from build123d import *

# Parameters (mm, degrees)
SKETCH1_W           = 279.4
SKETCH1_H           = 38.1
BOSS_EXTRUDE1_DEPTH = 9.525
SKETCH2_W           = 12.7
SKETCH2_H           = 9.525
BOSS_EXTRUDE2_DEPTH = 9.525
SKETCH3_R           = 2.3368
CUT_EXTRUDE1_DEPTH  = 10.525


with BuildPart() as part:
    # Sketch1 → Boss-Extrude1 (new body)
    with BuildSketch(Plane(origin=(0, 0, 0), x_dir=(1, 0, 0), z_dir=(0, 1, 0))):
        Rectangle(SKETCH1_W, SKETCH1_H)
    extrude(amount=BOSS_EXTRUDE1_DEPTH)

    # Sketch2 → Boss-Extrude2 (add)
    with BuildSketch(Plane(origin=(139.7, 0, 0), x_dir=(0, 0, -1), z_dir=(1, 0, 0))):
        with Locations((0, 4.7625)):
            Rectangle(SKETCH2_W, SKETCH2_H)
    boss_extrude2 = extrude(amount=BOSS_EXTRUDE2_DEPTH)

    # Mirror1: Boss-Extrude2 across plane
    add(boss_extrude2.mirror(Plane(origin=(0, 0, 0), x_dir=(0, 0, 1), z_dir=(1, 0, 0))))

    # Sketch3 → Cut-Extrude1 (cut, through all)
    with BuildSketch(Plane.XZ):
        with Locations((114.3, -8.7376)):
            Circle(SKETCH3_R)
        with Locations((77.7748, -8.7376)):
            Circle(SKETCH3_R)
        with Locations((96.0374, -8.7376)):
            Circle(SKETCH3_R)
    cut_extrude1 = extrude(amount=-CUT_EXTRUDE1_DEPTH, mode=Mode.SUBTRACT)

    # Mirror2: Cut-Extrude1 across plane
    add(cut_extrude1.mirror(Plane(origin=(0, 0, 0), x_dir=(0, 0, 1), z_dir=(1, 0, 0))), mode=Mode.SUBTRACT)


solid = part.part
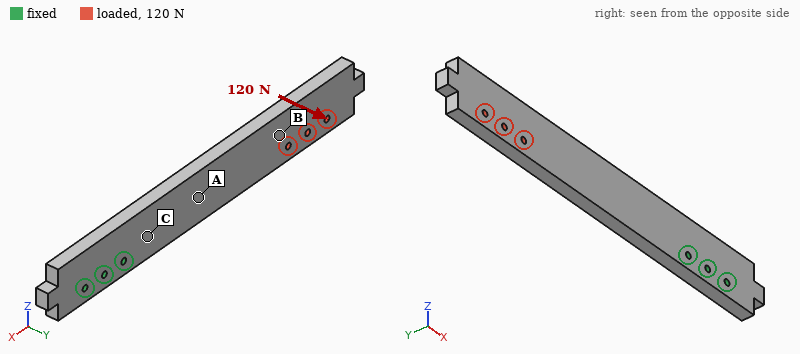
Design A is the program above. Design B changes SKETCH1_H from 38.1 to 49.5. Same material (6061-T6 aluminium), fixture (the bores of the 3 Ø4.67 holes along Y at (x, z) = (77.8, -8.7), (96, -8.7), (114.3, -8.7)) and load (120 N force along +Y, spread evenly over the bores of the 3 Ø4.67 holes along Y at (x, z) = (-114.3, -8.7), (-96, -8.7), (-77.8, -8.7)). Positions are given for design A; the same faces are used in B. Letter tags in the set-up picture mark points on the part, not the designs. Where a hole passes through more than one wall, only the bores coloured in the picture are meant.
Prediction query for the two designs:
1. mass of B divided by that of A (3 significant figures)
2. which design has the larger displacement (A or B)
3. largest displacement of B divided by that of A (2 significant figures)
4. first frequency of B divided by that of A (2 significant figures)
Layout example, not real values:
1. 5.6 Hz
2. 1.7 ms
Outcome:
1. 1.30
2. A
3. 0.78
4. 1.0
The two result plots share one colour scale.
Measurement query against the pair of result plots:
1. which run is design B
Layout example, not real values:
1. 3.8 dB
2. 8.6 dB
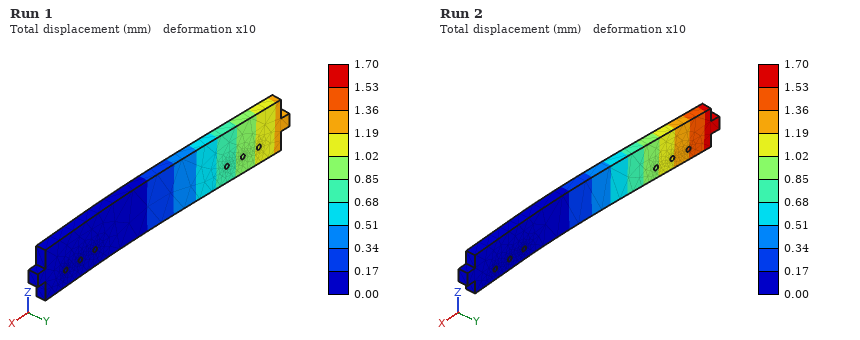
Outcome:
1. Run 1
